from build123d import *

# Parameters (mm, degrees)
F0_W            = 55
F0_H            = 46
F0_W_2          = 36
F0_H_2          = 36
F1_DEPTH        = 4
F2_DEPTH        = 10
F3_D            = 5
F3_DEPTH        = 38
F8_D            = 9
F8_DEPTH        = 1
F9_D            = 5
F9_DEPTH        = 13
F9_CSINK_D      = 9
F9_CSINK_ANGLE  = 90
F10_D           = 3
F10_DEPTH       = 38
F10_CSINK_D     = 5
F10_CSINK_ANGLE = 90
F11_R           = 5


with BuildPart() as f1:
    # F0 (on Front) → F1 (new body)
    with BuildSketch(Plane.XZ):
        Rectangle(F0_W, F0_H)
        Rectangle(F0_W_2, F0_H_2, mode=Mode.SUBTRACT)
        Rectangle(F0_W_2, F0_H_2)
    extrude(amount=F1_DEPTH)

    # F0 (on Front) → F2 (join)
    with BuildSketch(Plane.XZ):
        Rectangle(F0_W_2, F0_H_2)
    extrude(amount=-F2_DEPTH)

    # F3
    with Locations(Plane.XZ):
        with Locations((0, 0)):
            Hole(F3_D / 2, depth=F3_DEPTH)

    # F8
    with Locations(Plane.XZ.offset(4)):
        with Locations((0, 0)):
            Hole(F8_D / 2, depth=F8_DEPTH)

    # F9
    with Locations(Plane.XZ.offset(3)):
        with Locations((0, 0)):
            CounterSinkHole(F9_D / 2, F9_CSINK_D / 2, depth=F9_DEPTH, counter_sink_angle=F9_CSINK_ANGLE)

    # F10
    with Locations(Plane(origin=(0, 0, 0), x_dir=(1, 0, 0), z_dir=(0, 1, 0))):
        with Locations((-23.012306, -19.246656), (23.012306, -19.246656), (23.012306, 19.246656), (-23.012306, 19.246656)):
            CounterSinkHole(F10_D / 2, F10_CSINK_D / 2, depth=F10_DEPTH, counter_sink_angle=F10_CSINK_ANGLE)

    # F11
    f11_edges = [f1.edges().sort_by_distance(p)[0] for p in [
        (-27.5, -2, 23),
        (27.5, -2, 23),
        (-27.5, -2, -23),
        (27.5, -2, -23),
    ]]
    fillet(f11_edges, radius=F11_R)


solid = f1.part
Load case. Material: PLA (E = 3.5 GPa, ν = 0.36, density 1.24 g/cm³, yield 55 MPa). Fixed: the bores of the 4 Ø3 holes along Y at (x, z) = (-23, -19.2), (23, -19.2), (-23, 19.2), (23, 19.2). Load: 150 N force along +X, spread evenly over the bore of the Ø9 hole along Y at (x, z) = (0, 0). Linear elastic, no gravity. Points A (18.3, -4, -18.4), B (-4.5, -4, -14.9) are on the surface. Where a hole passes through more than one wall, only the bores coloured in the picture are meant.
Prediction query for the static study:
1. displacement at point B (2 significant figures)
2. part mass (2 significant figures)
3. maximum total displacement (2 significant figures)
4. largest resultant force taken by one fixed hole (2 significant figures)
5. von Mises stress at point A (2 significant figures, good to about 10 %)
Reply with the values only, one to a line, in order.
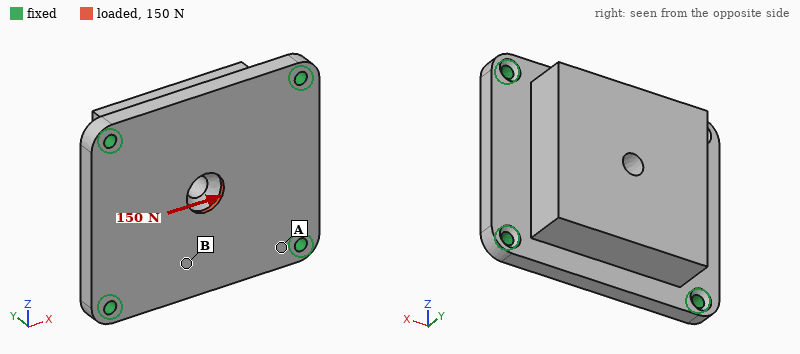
4.2 µm
28 g
10 µm
40 N
1.3 MPa
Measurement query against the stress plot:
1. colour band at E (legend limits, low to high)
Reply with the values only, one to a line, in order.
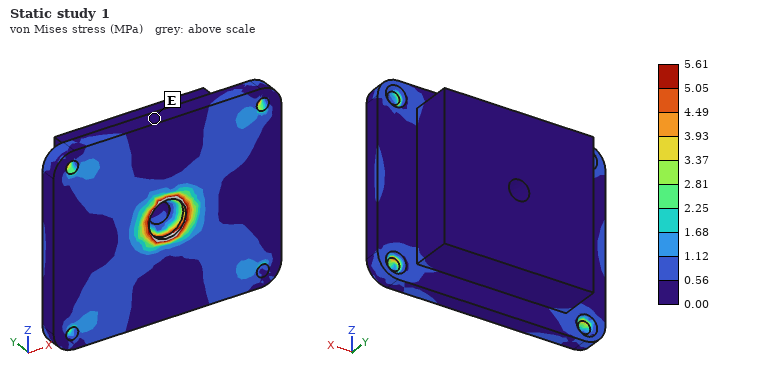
0.00 to 0.56 MPa
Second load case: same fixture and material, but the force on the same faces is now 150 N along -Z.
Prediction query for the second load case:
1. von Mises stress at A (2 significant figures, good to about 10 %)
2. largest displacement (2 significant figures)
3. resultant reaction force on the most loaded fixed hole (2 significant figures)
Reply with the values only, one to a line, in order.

0.92 MPa
12 µm
41 N
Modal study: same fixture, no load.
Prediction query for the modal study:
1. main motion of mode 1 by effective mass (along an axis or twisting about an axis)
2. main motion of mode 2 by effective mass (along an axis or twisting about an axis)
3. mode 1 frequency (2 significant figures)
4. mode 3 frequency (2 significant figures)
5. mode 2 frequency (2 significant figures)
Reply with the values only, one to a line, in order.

along Y
along Z
2800 Hz
4600 Hz
4000 Hz
